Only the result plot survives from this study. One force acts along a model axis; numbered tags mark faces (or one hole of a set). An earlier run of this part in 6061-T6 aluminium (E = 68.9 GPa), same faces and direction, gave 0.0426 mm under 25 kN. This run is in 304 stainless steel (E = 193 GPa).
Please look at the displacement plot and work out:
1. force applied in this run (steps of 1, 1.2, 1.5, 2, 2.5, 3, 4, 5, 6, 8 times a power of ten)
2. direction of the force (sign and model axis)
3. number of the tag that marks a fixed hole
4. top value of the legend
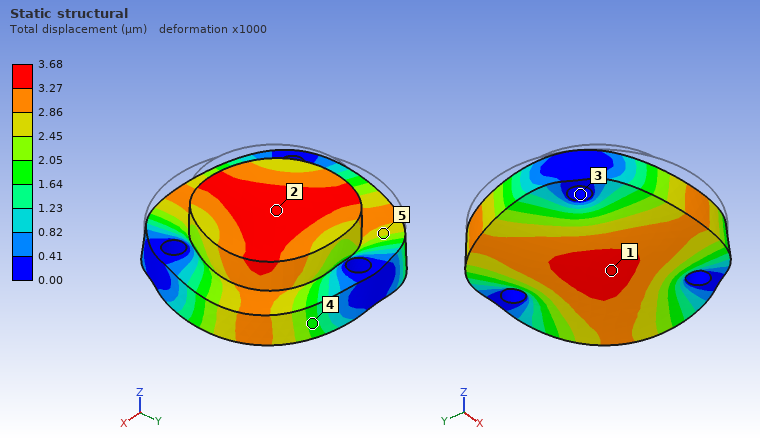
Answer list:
6 kN
-Z
3
3.68 µm
